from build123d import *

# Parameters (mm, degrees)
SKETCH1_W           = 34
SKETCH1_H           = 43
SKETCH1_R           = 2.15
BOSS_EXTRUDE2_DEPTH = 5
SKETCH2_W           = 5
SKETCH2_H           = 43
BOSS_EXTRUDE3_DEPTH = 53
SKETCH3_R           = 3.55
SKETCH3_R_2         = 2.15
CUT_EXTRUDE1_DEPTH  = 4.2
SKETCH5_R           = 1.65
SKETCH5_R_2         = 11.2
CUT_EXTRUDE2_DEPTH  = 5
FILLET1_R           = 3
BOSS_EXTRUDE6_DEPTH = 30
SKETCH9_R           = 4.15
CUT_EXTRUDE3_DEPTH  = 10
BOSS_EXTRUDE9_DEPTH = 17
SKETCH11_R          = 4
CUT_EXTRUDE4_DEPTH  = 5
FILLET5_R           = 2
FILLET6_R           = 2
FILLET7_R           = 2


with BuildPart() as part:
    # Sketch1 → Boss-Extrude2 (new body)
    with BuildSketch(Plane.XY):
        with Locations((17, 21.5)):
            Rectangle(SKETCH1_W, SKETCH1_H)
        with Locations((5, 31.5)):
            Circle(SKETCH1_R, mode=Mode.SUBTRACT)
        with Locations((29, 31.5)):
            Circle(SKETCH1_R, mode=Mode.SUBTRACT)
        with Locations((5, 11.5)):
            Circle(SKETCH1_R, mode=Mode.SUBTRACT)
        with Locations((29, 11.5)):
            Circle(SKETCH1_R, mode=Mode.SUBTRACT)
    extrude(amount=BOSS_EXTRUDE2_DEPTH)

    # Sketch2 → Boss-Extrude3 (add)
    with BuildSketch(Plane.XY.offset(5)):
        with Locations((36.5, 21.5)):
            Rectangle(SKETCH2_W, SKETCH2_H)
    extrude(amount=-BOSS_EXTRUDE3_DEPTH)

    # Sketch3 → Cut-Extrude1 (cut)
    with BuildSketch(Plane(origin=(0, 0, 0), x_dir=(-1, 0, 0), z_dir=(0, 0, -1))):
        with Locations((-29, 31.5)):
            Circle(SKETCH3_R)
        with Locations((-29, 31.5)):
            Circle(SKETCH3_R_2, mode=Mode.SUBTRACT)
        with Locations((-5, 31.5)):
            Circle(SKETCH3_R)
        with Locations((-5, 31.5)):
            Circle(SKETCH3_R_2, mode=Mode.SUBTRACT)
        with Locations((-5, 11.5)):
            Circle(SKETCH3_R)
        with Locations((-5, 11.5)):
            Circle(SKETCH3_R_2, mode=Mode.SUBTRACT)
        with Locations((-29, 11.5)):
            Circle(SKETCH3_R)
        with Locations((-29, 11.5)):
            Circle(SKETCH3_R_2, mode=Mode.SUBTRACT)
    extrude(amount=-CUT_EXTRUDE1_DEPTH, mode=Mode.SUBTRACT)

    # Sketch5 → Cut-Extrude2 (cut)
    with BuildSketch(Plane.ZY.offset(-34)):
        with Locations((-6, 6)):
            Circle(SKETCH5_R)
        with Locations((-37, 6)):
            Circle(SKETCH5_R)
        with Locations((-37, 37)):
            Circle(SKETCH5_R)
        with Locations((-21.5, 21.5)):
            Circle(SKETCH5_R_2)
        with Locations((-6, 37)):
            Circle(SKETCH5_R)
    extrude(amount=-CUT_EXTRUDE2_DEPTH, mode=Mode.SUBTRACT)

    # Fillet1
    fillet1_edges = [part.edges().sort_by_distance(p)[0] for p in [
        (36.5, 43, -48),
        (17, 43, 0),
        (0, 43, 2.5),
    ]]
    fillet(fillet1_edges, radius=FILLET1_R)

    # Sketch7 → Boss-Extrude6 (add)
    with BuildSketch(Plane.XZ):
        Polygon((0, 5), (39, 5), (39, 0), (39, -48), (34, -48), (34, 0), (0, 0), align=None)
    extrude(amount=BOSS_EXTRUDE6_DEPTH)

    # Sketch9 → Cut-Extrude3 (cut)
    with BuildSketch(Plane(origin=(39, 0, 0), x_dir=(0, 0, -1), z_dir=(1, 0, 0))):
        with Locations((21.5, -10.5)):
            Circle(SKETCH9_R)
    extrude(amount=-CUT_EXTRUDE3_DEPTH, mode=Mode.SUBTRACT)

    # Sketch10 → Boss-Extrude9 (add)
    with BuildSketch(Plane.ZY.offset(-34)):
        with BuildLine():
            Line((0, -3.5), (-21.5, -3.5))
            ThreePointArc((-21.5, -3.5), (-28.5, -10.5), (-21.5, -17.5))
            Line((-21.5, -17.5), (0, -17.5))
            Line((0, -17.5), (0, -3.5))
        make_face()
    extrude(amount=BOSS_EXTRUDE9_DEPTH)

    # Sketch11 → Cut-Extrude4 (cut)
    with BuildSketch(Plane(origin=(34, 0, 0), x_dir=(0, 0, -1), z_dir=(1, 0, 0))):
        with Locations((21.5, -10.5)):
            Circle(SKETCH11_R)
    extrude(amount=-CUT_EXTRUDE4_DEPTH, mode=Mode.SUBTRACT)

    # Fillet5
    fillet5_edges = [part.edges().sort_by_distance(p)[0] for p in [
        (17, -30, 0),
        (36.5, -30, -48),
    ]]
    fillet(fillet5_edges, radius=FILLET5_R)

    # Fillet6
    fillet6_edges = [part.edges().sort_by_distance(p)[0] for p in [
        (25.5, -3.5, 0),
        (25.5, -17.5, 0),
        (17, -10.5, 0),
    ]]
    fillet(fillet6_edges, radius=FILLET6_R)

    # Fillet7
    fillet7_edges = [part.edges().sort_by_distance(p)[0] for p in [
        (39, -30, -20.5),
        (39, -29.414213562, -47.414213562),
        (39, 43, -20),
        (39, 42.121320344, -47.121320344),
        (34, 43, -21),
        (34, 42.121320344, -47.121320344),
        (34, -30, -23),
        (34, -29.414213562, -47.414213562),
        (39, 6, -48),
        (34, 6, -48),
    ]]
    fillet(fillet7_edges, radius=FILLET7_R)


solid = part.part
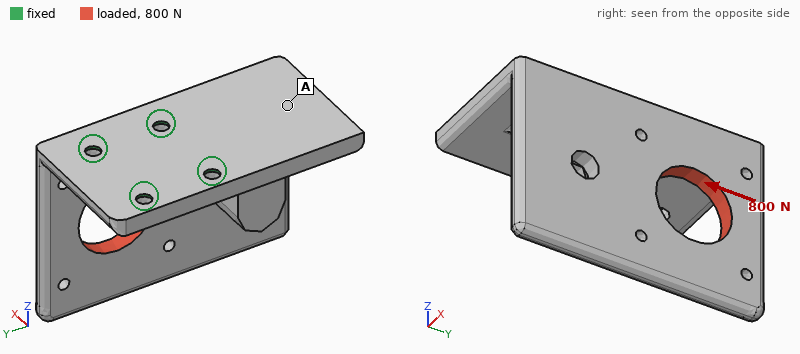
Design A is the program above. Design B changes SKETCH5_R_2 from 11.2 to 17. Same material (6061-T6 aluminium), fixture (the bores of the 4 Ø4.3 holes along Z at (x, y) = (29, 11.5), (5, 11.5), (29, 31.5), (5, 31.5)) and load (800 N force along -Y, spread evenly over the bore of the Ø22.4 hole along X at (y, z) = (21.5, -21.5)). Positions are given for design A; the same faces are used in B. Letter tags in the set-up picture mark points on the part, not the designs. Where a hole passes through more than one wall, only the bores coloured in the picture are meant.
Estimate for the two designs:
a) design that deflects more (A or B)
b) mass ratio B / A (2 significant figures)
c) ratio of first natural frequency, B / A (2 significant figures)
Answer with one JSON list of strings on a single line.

["B", "0.93", "0.96"]
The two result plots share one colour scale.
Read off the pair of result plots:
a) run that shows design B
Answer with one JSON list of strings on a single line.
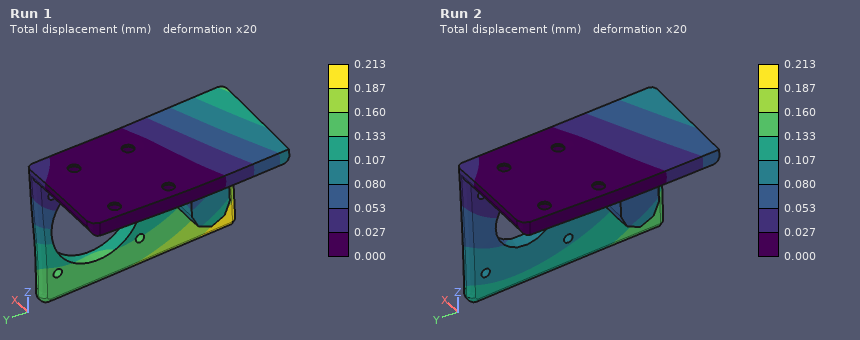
["Run 1"]
